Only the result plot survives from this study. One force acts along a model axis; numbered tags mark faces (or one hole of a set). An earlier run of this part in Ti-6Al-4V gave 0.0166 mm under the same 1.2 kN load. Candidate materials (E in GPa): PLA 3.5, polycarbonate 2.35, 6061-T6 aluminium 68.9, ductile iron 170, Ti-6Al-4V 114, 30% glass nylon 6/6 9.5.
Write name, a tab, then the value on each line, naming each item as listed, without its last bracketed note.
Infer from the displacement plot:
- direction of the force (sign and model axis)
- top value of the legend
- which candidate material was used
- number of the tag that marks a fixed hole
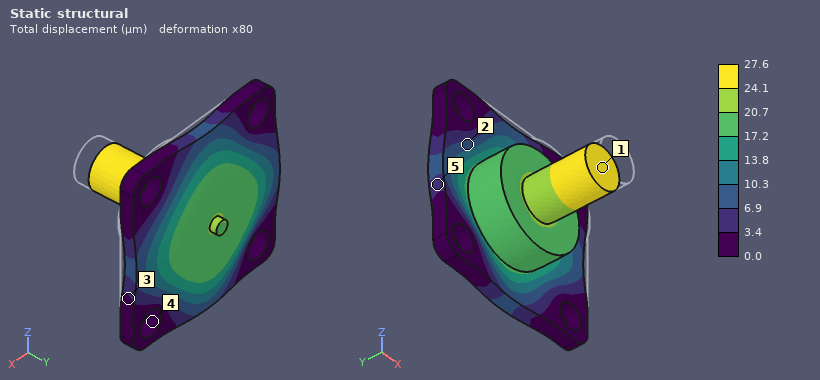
direction of the force	+Y
top value of the legend	27.6 µm
which candidate material was used	6061-T6 aluminium
number of the tag that marks a fixed hole	4
